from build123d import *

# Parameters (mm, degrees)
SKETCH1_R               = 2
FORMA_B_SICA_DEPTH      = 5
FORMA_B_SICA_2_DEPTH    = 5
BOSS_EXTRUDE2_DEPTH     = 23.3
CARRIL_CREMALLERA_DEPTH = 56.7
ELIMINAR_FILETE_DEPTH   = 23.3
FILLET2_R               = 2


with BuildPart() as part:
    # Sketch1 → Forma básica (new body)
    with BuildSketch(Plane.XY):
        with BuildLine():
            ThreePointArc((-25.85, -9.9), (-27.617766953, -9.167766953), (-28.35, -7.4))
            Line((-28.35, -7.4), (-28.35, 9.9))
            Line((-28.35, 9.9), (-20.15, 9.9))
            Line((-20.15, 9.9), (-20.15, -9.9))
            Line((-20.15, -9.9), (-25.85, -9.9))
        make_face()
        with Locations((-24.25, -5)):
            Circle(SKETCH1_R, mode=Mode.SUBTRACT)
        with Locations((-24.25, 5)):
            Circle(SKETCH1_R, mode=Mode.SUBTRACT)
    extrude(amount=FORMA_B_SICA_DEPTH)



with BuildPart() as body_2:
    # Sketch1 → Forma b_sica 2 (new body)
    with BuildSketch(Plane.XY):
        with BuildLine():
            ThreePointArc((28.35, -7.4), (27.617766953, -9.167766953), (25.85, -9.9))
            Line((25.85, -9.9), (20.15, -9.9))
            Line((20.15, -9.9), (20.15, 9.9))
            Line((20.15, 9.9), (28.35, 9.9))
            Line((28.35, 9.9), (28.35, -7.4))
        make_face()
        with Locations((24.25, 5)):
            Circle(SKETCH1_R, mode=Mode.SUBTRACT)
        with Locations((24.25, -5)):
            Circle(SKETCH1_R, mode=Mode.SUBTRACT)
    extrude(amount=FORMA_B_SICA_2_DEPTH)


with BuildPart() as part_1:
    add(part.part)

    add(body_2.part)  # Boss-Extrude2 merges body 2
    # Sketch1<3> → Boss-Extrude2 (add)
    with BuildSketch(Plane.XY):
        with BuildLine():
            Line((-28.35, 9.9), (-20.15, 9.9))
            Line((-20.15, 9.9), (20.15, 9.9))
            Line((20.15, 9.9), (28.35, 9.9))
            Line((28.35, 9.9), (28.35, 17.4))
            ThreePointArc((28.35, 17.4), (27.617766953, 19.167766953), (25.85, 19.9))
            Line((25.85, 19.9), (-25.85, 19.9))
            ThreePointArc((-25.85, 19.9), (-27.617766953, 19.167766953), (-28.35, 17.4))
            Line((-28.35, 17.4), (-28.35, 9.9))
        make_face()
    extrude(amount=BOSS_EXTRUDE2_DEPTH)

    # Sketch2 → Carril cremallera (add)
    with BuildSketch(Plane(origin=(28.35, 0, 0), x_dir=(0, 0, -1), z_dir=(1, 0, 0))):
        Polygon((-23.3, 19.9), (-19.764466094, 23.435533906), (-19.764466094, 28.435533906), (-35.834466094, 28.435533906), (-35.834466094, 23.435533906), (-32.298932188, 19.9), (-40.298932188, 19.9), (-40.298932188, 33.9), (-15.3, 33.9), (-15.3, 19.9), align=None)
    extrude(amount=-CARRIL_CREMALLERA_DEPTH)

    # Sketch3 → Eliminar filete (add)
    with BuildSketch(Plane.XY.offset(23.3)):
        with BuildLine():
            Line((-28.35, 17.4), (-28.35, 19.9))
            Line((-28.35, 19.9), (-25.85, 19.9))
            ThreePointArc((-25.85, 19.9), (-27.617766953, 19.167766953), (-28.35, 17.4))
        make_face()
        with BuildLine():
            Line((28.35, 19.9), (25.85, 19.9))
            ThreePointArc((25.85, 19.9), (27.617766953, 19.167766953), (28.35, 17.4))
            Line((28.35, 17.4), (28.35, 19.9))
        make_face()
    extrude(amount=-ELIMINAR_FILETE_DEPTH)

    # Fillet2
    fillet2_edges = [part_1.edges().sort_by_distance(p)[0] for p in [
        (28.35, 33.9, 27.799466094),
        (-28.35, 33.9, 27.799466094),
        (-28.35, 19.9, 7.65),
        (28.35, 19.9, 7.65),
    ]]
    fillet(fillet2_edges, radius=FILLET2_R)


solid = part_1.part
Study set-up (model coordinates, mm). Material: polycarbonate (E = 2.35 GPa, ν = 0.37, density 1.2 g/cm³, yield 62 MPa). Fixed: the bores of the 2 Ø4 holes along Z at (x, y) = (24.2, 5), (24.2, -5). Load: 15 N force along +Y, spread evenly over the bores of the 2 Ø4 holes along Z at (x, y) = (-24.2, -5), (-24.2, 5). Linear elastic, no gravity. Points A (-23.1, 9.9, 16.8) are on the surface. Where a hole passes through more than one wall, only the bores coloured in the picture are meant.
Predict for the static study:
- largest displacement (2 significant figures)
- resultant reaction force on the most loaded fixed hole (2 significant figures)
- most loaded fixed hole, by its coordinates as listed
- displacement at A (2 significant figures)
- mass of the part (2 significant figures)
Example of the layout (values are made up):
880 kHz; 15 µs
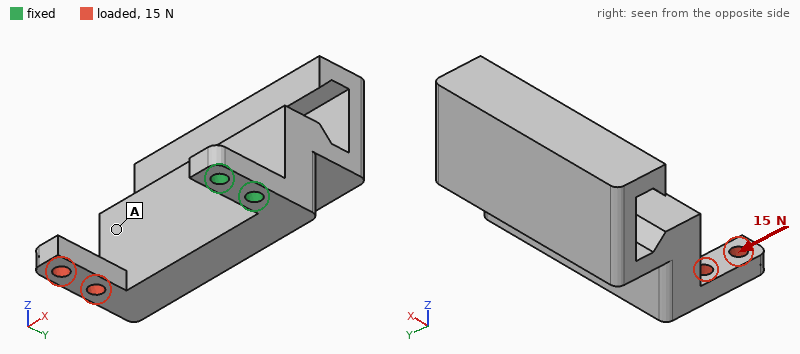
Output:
0.78 mm; 21 N; (24.2, 5); 0.65 mm; 33 g
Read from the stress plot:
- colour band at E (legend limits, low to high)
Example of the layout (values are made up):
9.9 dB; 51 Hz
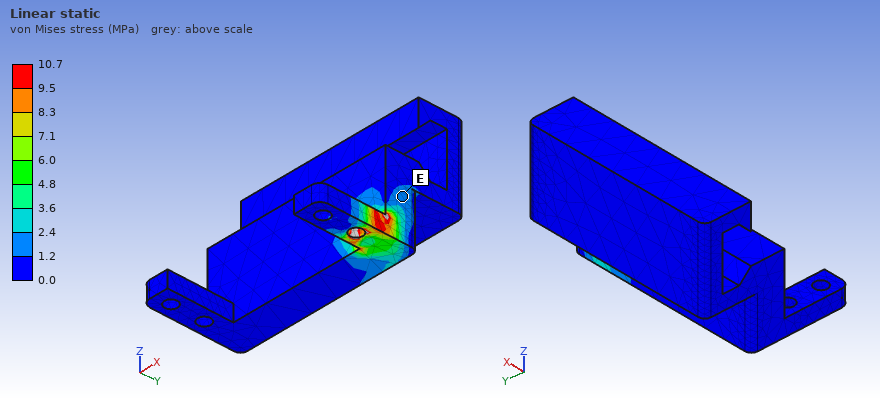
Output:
1.2 to 2.4 MPa
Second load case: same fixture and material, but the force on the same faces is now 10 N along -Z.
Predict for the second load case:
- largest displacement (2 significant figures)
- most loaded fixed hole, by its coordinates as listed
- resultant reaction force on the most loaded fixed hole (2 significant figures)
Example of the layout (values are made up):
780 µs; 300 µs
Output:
0.87 mm; (24.2, 5); 9.6 N
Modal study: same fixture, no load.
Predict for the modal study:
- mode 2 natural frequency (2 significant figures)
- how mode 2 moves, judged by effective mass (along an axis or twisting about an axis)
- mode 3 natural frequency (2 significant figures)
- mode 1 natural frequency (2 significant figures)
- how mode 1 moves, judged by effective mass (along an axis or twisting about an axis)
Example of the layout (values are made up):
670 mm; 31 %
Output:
170 Hz; along Y; 330 Hz; 140 Hz; along Z
